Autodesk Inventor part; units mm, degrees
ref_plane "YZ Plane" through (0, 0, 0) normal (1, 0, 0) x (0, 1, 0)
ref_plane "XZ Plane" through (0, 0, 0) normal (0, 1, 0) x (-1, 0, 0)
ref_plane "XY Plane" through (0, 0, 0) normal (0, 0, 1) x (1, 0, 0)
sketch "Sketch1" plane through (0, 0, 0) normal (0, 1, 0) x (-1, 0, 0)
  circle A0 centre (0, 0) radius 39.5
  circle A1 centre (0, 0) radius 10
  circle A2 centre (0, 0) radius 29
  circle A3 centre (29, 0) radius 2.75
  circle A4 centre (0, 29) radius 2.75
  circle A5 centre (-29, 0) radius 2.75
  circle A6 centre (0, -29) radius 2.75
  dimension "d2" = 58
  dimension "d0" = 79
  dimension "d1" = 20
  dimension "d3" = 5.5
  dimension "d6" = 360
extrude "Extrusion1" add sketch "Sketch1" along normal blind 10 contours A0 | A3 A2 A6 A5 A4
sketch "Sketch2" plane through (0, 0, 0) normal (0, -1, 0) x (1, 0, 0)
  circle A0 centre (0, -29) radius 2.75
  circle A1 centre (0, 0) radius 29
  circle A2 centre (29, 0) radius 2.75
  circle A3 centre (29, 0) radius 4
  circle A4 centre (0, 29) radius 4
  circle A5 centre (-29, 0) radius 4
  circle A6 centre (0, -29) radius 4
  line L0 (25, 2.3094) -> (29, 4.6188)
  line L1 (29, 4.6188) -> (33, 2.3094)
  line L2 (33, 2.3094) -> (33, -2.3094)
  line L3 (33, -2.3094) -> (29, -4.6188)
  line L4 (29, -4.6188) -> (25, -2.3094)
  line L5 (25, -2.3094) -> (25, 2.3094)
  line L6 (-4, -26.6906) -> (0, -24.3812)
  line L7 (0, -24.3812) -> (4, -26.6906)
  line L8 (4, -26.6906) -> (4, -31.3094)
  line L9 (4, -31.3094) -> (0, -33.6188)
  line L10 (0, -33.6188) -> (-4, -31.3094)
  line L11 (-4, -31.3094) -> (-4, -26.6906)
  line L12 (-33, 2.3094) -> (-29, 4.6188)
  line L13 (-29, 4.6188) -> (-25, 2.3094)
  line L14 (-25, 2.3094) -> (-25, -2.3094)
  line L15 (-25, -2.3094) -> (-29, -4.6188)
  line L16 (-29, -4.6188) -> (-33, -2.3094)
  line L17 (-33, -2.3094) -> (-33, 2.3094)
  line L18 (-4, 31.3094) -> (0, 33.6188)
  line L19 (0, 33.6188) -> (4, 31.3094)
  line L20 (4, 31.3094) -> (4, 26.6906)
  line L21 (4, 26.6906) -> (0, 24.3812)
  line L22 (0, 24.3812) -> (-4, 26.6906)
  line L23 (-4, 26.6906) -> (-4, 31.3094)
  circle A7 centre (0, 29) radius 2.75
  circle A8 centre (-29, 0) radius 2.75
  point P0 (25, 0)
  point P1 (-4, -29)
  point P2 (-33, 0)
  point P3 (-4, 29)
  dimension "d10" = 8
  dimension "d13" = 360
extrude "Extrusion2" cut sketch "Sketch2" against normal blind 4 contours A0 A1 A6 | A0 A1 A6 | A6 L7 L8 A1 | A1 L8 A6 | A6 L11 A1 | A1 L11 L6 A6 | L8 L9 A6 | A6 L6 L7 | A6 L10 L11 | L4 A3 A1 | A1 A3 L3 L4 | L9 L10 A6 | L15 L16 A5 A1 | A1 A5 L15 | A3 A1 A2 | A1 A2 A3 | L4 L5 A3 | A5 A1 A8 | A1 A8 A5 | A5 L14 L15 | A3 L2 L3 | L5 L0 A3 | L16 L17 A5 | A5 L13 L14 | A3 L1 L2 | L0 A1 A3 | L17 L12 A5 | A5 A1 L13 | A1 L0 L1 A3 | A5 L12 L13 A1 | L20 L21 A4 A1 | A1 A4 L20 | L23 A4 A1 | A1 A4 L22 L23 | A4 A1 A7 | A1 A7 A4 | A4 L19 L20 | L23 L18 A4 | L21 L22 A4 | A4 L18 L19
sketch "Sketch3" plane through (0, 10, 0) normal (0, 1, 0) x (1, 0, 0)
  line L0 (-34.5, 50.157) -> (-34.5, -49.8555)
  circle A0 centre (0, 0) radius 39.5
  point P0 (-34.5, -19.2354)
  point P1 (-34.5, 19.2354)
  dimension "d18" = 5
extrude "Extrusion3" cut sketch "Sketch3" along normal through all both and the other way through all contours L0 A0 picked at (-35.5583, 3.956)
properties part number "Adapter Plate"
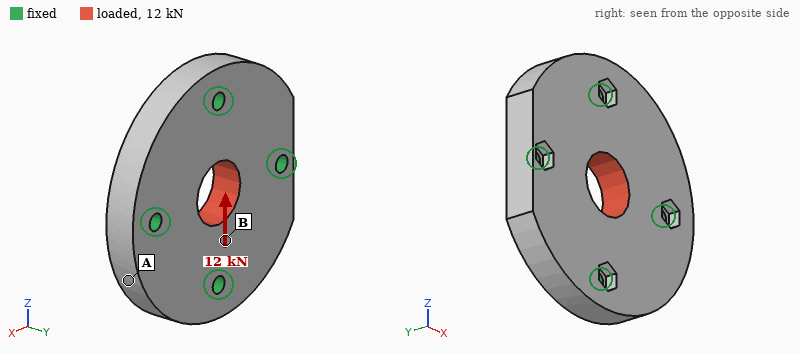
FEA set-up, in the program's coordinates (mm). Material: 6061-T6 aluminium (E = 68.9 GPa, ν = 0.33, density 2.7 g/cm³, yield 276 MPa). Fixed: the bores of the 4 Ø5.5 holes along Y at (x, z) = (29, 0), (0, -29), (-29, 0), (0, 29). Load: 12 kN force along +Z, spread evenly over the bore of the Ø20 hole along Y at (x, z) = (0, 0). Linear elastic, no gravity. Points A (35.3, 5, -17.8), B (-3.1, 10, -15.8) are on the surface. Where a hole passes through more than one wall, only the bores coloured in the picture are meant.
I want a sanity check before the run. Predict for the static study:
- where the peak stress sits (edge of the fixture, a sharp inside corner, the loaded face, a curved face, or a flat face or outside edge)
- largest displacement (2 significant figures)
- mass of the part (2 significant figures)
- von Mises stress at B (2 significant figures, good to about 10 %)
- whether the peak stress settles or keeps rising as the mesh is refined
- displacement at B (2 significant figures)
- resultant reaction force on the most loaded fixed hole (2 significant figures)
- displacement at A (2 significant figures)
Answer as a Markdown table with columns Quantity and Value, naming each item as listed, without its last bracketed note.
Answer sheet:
| Quantity | Value |
|---|---|
| where the peak stress sits | edge of the fixture |
| largest displacement | 8.6 µm |
| mass of the part | 120 g |
| von Mises stress at B | 24 MPa |
| whether the peak stress settles or keeps rising as the mesh is refined | keeps rising |
| displacement at B | 5.1 µm |
| resultant reaction force on the most loaded fixed hole | 3.7 kN |
| displacement at A | 3.1 µm |
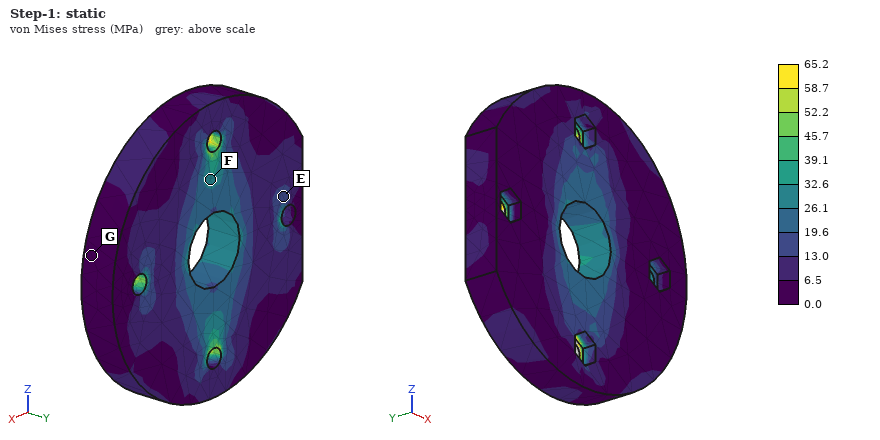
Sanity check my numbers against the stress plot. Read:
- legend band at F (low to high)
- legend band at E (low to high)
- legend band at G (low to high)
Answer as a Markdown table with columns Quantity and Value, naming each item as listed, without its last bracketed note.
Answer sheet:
| Quantity | Value |
|---|---|
| legend band at F | 26.1 to 32.6 MPa |
| legend band at E | 13.0 to 19.6 MPa |
| legend band at G | 0.0 to 6.5 MPa |
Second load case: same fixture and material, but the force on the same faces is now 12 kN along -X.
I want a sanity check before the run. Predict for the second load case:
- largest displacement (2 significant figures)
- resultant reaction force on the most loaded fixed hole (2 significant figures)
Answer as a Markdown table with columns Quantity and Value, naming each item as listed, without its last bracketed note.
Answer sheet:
| Quantity | Value |
|---|---|
| largest displacement | 8.6 µm |
| resultant reaction force on the most loaded fixed hole | 3.7 kN |
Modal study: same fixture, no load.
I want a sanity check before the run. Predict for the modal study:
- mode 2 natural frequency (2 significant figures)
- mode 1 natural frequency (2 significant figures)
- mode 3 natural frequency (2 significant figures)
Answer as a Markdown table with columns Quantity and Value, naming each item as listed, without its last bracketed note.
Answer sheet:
| Quantity | Value |
|---|---|
| mode 2 natural frequency | 13 kHz |
| mode 1 natural frequency | 12 kHz |
| mode 3 natural frequency | 14 kHz |
